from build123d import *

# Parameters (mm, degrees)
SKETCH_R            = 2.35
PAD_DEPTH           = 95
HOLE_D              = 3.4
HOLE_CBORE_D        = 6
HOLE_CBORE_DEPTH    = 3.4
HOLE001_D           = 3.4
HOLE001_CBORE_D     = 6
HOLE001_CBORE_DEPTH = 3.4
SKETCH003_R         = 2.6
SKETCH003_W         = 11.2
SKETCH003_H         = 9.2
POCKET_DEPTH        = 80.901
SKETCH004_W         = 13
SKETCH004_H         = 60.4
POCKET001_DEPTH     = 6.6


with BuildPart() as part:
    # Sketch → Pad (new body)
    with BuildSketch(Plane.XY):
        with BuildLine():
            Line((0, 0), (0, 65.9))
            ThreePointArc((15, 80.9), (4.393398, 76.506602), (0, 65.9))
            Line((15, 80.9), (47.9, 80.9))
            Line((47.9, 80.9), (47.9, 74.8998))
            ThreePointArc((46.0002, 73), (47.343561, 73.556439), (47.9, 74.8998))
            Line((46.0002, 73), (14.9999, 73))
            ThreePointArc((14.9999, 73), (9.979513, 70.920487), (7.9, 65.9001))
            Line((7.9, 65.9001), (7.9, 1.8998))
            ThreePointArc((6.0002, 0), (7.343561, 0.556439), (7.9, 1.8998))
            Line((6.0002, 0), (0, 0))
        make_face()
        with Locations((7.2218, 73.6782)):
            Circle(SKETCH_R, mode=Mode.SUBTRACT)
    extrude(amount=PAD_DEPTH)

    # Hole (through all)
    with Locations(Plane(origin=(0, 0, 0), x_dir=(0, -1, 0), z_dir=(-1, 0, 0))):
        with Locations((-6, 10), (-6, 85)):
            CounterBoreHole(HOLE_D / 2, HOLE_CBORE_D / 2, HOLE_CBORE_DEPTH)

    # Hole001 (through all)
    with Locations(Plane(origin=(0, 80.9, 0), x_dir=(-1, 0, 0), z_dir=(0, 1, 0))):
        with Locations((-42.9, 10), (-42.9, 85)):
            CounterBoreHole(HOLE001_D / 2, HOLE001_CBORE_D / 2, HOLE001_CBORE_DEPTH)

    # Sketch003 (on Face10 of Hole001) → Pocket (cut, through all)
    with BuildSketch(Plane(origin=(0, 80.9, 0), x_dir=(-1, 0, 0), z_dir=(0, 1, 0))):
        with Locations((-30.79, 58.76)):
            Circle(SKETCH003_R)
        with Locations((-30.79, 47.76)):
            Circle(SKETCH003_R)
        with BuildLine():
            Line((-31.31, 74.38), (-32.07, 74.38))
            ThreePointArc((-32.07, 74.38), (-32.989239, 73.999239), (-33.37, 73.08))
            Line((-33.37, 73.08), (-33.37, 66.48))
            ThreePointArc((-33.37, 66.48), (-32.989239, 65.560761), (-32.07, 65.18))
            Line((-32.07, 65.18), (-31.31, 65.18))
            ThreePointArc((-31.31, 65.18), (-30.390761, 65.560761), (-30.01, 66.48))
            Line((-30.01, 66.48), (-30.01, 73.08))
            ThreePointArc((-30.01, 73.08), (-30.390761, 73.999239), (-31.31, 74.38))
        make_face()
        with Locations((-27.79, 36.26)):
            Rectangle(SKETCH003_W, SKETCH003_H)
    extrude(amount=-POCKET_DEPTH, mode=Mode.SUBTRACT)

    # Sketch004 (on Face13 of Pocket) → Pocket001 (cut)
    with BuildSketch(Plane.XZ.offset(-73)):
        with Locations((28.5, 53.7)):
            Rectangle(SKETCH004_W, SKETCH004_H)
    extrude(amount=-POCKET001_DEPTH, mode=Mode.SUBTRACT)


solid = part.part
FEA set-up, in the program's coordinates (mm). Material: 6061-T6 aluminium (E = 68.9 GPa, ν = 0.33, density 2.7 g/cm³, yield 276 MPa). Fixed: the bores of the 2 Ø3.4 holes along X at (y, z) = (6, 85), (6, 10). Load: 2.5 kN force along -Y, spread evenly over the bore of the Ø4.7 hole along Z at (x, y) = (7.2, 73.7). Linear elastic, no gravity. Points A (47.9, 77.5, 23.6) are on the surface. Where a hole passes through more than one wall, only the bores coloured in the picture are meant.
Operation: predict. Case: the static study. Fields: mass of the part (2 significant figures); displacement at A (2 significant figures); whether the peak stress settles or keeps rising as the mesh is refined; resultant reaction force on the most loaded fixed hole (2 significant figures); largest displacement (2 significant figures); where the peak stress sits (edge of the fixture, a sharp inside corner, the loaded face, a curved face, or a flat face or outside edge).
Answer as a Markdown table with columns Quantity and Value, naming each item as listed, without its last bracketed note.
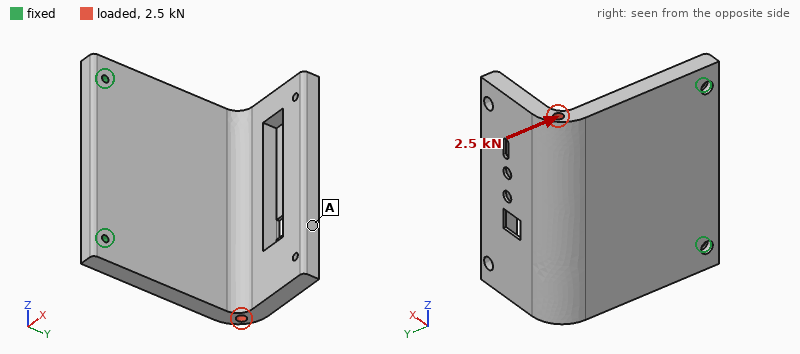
| Quantity | Value |
|---|---|
| mass of the part | 210 g |
| displacement at A | 0.17 mm |
| whether the peak stress settles or keeps rising as the mesh is refined | keeps rising |
| resultant reaction force on the most loaded fixed hole | 1.3 kN |
| largest displacement | 0.18 mm |
| where the peak stress sits | edge of the fixture |
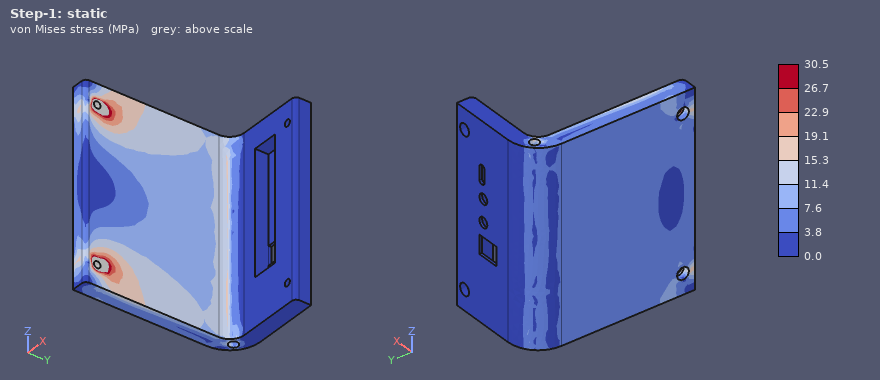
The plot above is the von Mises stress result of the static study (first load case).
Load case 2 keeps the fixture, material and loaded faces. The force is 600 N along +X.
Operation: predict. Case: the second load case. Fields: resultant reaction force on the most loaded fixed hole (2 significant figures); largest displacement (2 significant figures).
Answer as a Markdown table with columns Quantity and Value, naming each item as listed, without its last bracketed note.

| Quantity | Value |
|---|---|
| resultant reaction force on the most loaded fixed hole | 310 N |
| largest displacement | 0.86 mm |
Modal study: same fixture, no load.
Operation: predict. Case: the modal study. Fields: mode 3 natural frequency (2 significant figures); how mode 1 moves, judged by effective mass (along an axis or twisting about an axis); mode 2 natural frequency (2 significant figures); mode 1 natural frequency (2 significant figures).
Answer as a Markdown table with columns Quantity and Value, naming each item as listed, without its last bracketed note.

| Quantity | Value |
|---|---|
| mode 3 natural frequency | 1900 Hz |
| how mode 1 moves, judged by effective mass | along X |
| mode 2 natural frequency | 1200 Hz |
| mode 1 natural frequency | 430 Hz |
